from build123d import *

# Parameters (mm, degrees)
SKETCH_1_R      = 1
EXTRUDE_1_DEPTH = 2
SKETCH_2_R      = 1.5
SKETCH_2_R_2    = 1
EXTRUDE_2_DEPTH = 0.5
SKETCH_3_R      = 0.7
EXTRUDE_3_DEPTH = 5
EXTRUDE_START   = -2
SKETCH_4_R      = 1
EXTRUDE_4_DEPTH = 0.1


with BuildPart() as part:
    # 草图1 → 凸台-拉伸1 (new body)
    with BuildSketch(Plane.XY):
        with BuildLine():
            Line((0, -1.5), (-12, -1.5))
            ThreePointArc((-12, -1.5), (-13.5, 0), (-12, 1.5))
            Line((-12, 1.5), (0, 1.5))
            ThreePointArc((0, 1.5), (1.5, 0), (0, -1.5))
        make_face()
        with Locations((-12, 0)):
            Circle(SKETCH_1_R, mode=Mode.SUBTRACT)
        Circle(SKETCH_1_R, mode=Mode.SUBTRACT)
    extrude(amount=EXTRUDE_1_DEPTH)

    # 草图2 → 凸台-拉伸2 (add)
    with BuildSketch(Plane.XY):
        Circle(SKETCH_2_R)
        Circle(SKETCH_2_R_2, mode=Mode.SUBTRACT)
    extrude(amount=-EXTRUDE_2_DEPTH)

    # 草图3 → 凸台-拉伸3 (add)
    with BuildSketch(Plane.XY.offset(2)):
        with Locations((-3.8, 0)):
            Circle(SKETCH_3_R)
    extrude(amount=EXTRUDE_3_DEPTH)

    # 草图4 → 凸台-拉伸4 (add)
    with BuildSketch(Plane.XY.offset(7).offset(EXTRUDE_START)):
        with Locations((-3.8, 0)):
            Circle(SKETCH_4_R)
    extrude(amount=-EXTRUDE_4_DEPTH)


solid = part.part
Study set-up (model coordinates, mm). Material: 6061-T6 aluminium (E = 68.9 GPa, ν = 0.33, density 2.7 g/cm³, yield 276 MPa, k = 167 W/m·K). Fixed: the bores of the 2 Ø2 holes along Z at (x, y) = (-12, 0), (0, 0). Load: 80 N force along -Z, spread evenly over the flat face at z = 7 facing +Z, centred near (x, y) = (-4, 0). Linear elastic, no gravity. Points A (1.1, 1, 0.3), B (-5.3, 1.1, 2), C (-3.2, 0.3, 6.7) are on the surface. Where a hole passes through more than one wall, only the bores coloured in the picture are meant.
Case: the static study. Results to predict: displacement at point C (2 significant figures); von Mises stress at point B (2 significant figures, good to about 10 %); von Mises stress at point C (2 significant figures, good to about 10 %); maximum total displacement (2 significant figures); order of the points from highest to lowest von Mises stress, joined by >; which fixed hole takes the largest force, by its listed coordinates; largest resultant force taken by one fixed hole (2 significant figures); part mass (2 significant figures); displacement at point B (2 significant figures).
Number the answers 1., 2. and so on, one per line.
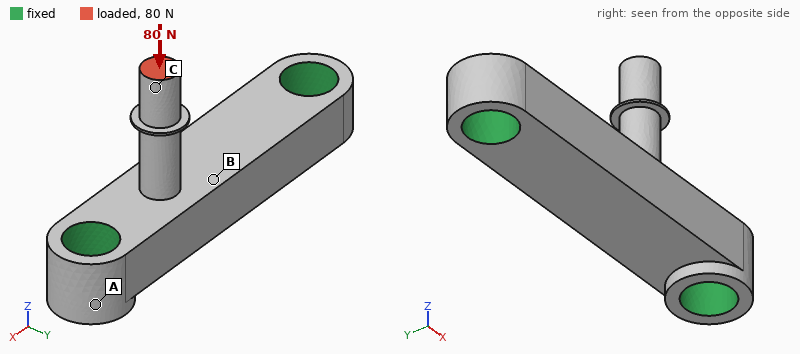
1. 6.9 µm
2. 24 MPa
3. 52 MPa
4. 8.1 µm
5. C > B > A
6. (0, 0)
7. 63 N
8. 0.23 g
9. 3.0 µm
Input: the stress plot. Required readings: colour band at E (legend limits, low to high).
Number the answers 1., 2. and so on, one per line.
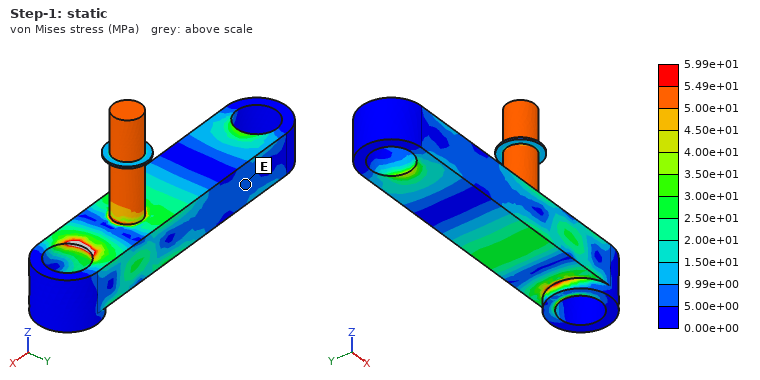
1. 5.00e+00 to 9.99e+00 MPa
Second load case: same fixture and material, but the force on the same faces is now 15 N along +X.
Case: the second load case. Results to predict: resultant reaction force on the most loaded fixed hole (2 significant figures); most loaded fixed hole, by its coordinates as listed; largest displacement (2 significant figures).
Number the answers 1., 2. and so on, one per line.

1. 15 N
2. (0, 0)
3. 63 µm
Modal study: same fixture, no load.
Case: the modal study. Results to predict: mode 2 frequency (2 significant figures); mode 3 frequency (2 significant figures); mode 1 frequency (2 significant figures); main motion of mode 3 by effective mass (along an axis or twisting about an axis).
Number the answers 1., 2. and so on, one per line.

1. 33 kHz
2. 75 kHz
3. 31 kHz
4. along Z
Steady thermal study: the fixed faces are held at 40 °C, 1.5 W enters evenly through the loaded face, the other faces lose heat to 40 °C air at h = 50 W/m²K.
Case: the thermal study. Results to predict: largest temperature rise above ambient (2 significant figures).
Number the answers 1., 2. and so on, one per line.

1. 34 K
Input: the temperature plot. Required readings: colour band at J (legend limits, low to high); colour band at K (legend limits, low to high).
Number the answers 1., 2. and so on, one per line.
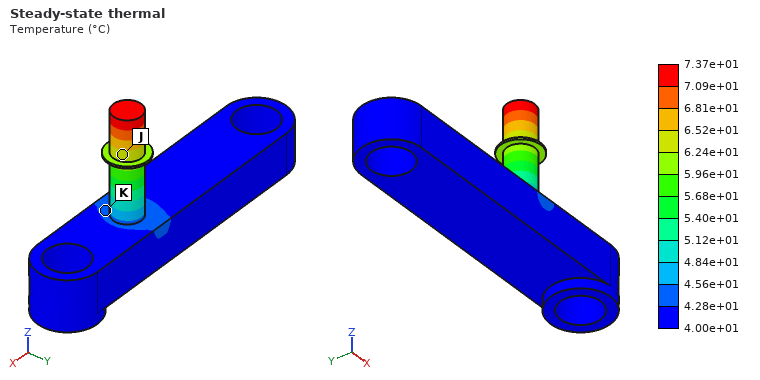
1. 6.24e+01 to 6.52e+01 °C
2. 4.28e+01 to 4.56e+01 °C
